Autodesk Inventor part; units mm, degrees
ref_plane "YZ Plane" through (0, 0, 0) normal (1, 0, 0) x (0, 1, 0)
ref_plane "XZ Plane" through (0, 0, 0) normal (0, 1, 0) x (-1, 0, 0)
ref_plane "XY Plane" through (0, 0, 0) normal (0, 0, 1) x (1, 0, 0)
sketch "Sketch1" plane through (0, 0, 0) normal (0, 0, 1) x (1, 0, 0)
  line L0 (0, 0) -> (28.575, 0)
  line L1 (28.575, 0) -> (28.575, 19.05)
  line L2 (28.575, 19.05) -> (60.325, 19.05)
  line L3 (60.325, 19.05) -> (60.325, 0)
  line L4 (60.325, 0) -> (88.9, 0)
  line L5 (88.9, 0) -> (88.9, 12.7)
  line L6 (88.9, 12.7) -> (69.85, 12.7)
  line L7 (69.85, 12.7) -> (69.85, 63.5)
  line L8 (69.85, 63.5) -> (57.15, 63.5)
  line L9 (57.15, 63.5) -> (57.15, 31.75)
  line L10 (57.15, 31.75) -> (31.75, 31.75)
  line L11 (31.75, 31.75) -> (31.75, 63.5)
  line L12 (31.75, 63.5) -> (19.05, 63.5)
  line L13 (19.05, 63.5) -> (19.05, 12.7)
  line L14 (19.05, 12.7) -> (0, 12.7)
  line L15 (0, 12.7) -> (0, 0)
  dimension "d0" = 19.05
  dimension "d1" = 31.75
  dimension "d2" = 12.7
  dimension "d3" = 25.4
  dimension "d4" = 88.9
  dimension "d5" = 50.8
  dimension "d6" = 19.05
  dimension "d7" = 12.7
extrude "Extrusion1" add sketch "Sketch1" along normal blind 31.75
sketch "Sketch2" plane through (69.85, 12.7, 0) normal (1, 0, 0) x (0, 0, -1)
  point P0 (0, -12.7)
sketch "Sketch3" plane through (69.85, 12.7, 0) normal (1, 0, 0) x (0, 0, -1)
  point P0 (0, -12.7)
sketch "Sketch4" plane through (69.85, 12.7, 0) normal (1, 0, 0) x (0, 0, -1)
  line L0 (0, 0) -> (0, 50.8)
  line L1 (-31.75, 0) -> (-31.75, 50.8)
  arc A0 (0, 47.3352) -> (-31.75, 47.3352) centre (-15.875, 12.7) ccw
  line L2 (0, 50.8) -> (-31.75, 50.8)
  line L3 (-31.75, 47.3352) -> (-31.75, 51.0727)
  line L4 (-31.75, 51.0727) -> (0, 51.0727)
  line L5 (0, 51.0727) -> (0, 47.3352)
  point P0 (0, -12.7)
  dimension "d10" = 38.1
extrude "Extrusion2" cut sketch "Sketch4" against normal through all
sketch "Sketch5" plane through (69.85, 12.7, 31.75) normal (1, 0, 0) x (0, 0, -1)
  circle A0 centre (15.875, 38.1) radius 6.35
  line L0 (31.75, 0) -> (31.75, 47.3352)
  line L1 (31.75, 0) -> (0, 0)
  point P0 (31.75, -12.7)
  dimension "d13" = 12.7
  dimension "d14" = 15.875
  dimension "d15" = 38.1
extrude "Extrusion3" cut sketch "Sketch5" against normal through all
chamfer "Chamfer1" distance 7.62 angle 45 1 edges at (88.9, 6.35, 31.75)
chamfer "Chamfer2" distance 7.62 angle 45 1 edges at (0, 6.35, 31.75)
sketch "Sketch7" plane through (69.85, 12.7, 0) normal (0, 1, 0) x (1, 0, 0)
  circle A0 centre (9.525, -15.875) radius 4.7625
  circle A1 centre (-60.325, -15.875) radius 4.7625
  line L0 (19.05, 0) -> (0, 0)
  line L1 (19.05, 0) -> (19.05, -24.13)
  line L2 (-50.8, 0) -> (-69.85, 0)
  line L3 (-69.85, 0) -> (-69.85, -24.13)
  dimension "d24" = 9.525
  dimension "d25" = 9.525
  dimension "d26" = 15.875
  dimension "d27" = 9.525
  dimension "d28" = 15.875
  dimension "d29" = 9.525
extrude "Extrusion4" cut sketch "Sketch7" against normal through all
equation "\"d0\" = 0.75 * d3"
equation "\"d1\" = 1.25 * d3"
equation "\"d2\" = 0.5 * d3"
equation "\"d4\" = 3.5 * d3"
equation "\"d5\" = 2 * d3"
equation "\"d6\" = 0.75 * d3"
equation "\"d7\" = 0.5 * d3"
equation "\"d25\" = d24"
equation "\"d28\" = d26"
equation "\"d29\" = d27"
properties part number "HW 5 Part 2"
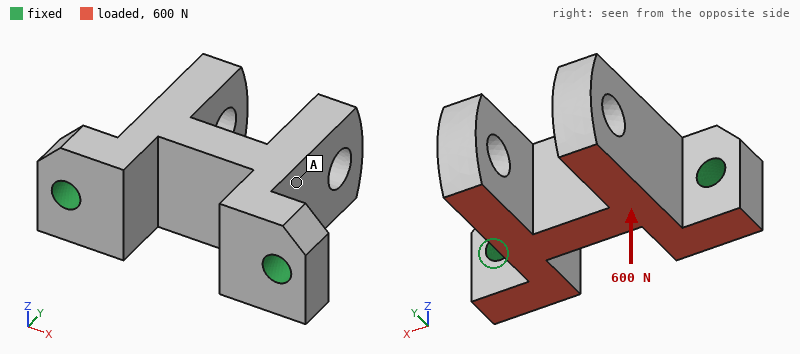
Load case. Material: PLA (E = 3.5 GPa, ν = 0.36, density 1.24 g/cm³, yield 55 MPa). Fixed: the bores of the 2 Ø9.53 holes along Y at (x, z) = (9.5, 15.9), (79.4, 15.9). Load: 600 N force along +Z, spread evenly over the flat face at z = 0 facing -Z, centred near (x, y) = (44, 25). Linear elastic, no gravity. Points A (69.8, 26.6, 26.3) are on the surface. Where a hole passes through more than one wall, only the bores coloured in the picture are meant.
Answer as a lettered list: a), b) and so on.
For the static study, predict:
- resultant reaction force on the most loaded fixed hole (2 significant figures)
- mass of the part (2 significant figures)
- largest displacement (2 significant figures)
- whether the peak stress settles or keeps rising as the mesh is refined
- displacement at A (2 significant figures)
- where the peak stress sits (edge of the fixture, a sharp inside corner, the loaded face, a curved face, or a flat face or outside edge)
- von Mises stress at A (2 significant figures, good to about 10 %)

a) 300 N
b) 82 g
c) 0.21 mm
d) keeps rising
e) 0.086 mm
f) edge of the fixture
g) 1.3 MPa
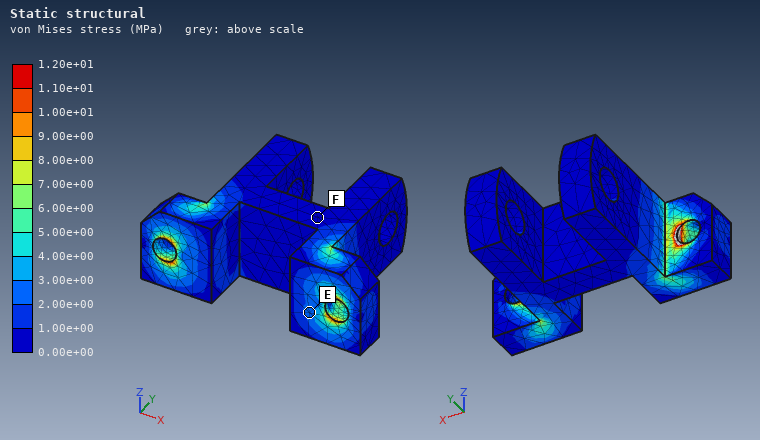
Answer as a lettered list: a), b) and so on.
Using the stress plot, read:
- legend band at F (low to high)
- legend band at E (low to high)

a) 0.00e+00 to 1.00e+00 MPa
b) 2.00e+00 to 3.00e+00 MPa
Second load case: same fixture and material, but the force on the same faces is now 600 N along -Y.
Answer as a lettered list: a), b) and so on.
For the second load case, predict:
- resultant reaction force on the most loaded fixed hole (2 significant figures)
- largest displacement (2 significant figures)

a) 320 N
b) 0.15 mm
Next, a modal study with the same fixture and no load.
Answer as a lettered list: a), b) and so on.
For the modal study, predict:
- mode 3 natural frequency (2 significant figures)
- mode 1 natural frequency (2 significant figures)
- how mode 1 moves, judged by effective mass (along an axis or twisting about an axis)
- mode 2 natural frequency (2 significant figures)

a) 1900 Hz
b) 1100 Hz
c) along Z
d) 1800 Hz
